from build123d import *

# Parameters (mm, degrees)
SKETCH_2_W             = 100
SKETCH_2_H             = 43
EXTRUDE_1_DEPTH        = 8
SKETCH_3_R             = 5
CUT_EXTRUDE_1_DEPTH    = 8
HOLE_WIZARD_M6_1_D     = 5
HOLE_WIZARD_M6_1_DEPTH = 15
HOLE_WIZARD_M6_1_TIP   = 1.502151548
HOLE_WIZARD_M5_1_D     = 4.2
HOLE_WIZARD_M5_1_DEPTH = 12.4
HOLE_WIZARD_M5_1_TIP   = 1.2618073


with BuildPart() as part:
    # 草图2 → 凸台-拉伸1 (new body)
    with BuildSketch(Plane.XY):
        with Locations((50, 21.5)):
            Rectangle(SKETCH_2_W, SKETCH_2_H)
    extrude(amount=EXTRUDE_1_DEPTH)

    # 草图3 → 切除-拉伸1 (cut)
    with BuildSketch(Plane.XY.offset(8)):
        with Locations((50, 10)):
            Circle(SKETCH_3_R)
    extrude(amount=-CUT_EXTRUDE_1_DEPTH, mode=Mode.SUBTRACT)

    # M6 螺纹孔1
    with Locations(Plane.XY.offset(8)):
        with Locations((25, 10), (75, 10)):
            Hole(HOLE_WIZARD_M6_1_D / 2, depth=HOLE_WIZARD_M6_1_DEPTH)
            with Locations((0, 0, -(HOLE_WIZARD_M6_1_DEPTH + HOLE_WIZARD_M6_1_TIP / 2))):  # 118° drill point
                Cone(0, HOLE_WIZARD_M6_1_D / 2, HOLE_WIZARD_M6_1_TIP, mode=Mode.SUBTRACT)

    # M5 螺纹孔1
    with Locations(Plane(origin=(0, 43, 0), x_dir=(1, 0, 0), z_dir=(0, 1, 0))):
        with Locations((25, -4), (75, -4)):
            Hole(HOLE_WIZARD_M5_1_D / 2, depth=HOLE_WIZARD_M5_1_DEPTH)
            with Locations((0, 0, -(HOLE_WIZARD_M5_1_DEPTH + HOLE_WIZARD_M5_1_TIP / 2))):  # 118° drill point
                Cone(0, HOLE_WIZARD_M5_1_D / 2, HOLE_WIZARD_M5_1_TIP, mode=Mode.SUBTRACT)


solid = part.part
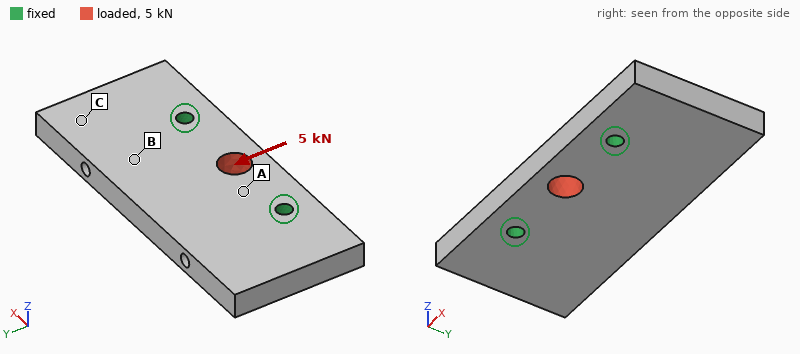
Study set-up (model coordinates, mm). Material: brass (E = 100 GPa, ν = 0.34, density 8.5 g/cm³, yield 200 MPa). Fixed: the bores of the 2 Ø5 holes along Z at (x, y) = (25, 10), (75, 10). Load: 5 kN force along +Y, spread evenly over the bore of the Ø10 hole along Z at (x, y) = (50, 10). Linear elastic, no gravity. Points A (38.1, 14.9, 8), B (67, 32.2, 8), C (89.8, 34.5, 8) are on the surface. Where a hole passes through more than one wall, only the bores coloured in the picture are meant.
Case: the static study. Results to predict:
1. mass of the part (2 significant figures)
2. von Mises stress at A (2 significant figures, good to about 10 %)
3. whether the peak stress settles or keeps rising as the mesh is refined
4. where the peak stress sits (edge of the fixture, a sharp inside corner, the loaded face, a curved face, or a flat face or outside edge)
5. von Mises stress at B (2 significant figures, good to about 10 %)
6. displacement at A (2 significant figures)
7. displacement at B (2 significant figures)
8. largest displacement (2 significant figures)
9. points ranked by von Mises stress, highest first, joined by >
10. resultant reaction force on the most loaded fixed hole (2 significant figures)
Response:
280 g
21 MPa
keeps rising
edge of the fixture
11 MPa
5.4 µm
3.9 µm
12 µm
A > B > C
2.6 kN
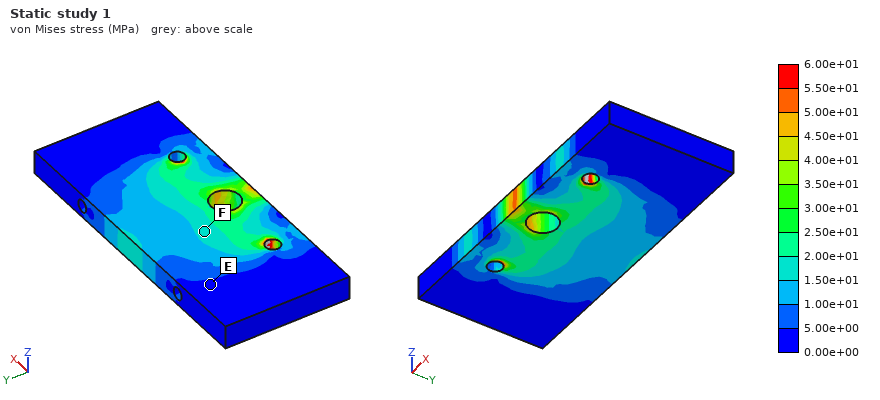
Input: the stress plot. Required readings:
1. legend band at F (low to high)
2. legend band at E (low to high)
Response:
1.50e+01 to 2.00e+01 MPa
0.00e+00 to 5.00e+00 MPa
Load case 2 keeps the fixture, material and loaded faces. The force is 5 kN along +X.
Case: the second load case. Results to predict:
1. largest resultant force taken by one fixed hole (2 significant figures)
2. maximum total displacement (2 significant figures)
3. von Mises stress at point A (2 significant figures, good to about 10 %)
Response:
2.5 kN
4.5 µm
15 MPa
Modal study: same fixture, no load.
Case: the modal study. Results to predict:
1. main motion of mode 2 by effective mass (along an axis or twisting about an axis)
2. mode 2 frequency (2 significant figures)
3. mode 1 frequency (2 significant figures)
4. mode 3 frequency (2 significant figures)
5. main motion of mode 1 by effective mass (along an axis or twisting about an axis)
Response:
twisting about Y
3600 Hz
3000 Hz
4600 Hz
along Z
